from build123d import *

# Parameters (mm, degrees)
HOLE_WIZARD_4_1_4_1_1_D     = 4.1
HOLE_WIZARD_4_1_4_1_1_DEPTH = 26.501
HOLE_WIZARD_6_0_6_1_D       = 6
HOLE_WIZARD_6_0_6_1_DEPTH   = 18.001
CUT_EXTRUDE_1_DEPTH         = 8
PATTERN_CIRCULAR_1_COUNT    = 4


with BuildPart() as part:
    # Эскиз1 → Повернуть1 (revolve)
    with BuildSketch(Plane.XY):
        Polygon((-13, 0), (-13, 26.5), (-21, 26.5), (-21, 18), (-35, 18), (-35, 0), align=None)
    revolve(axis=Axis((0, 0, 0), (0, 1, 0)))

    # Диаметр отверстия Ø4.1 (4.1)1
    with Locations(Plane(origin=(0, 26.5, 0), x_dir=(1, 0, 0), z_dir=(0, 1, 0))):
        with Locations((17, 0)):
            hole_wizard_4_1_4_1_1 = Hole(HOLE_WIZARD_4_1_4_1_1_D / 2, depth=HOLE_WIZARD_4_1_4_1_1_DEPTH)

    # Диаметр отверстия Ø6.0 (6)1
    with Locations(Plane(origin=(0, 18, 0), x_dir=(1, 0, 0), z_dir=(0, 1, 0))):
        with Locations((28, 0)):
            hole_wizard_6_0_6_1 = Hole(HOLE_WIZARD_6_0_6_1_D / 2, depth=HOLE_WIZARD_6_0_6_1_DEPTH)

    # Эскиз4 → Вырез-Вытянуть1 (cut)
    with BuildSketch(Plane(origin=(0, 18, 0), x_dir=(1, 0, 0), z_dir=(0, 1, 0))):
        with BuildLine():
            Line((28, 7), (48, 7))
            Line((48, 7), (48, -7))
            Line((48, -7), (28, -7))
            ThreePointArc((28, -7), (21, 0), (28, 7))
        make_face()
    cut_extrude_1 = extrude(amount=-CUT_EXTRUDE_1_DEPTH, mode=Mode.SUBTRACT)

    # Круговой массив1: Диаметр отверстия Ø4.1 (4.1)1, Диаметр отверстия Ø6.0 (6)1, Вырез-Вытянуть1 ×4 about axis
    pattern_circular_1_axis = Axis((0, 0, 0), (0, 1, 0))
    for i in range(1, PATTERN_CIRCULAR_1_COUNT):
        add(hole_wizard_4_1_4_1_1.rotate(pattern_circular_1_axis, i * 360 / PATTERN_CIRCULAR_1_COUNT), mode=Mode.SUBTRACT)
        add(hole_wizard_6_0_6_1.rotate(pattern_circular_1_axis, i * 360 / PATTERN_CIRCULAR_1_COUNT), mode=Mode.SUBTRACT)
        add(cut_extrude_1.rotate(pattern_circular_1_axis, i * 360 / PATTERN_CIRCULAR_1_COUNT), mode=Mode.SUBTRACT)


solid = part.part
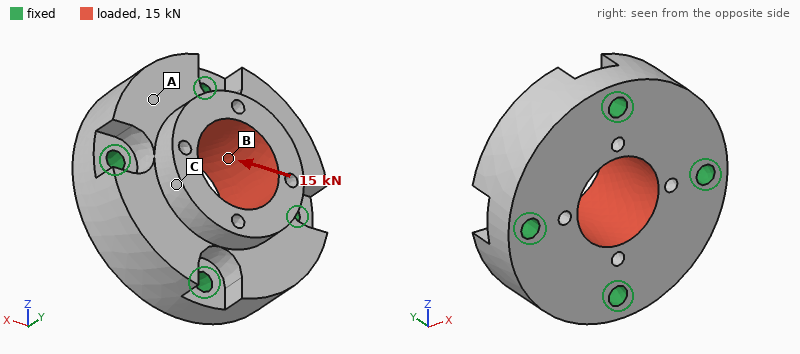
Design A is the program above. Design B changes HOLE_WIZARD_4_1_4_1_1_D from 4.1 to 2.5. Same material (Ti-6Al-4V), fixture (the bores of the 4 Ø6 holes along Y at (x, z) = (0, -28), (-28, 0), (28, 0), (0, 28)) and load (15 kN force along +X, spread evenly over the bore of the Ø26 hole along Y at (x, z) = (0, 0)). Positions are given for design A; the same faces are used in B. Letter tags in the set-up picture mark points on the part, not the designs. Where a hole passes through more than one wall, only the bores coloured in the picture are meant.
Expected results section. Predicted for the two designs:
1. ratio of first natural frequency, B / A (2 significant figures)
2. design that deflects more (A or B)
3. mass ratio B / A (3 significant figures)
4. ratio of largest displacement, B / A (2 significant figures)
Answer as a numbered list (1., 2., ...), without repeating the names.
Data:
1. 1.0
2. A
3. 1.01
4. 0.91
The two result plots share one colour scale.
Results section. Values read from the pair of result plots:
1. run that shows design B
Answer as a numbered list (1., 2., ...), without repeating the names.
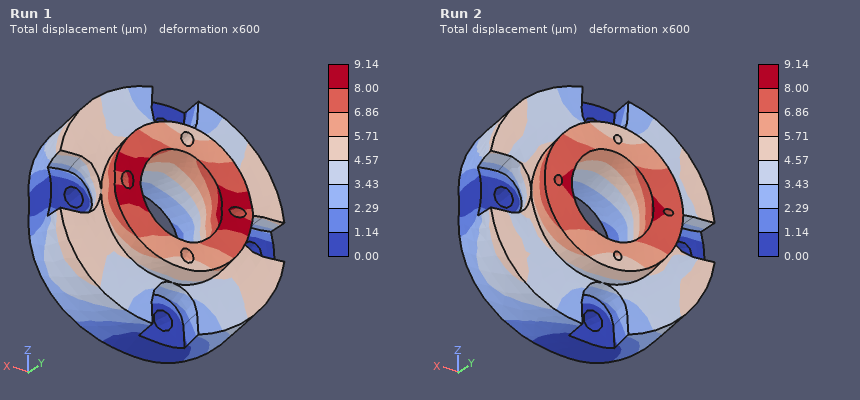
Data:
1. Run 2
